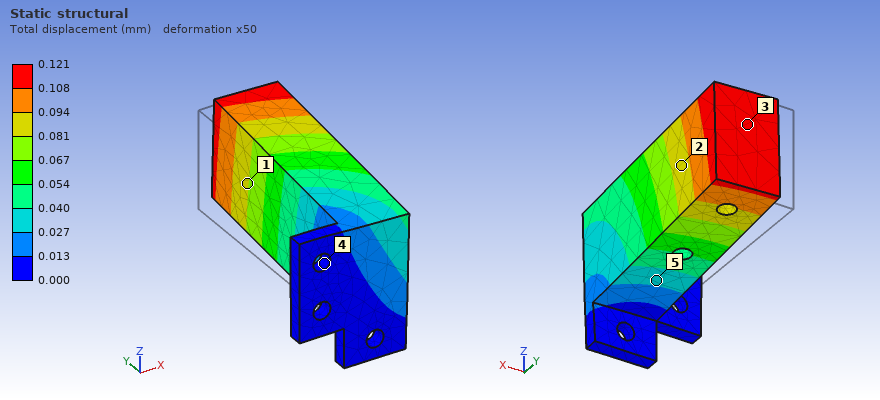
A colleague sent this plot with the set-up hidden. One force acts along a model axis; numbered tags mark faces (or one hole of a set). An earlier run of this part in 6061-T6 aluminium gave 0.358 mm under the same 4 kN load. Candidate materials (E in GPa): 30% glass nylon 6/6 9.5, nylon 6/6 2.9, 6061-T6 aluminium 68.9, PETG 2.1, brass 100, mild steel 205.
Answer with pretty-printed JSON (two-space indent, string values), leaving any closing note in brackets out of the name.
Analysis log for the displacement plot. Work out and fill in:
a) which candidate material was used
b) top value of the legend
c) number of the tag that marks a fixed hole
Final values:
{
  "which candidate material was used": "mild steel",
  "top value of the legend": "0.121 mm",
  "number of the tag that marks a fixed hole": "4"
}
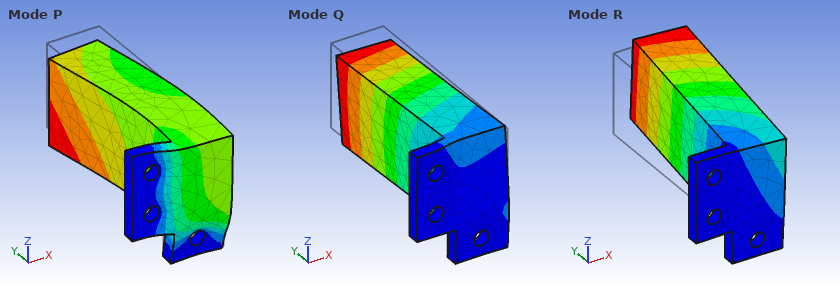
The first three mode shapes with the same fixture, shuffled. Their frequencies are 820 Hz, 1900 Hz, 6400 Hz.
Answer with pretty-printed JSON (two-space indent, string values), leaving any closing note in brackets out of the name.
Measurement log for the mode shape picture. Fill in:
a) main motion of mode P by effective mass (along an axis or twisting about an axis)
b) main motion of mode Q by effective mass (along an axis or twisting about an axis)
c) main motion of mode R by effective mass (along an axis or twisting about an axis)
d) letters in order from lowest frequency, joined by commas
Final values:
{
  "main motion of mode P by effective mass": "along Y",
  "main motion of mode Q by effective mass": "along Z",
  "main motion of mode R by effective mass": "along X",
  "letters in order from lowest frequency, joined by commas": "R, Q, P"
}
